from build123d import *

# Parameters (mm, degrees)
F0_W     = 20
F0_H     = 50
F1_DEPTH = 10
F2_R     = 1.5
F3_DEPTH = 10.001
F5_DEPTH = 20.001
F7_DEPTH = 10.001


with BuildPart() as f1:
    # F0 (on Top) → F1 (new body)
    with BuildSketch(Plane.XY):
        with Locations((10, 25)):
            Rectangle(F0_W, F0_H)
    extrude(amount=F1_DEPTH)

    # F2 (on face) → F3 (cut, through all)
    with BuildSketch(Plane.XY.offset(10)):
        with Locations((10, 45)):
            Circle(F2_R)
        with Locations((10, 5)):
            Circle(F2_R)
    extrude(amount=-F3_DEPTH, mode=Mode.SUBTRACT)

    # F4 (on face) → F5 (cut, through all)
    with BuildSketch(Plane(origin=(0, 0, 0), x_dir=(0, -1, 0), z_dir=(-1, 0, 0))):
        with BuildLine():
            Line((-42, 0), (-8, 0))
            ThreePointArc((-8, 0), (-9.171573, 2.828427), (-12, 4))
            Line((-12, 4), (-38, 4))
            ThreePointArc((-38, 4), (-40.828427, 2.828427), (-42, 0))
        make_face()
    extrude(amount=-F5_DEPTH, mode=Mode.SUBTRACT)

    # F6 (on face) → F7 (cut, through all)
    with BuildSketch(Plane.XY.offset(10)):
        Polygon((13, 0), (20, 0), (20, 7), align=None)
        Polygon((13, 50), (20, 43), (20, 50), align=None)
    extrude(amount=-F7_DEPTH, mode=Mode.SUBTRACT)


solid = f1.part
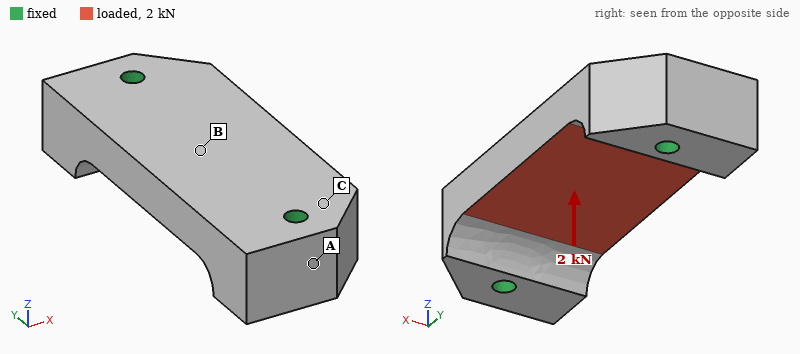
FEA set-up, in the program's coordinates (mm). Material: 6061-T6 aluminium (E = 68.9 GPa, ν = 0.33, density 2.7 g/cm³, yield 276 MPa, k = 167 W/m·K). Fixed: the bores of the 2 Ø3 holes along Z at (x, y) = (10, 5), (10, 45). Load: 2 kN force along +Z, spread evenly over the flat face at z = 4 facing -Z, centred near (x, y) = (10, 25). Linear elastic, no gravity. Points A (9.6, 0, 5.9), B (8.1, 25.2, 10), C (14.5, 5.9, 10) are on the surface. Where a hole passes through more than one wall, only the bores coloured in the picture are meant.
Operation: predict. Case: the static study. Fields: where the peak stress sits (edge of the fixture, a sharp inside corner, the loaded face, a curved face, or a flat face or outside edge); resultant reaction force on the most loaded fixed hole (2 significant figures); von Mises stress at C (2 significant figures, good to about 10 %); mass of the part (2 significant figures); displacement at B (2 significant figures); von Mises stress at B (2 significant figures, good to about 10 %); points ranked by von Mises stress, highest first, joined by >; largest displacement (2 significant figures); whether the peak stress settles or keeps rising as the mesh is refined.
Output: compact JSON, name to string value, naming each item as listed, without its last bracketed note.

{"where the peak stress sits": "edge of the fixture", "resultant reaction force on the most loaded fixed hole": "1.0 kN", "von Mises stress at C": "22 MPa", "mass of the part": "18 g", "displacement at B": "19 µm", "von Mises stress at B": "36 MPa", "points ranked by von Mises stress, highest first, joined by >": "B > C > A", "largest displacement": "22 µm", "whether the peak stress settles or keeps rising as the mesh is refined": "keeps rising"}
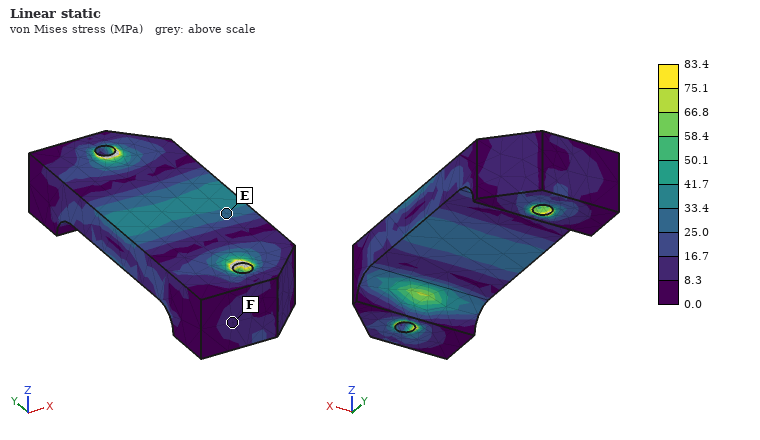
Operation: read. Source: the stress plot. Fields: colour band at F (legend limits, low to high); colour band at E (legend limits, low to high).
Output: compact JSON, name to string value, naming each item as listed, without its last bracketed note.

{"colour band at F": "8.3 to 16.7 MPa", "colour band at E": "25.0 to 33.4 MPa"}
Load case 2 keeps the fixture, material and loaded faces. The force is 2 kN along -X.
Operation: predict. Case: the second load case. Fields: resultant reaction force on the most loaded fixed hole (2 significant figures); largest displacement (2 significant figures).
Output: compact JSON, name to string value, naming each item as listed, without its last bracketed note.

{"resultant reaction force on the most loaded fixed hole": "1.0 kN", "largest displacement": "15 µm"}
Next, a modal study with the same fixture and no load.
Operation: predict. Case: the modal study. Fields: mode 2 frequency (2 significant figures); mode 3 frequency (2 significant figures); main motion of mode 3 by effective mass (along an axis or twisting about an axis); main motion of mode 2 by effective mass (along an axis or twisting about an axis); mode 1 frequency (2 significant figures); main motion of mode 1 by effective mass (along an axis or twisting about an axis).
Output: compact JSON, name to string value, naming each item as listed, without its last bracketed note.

{"mode 2 frequency": "23 kHz", "mode 3 frequency": "25 kHz", "main motion of mode 3 by effective mass": "along X", "main motion of mode 2 by effective mass": "along X", "mode 1 frequency": "19 kHz", "main motion of mode 1 by effective mass": "along Z"}
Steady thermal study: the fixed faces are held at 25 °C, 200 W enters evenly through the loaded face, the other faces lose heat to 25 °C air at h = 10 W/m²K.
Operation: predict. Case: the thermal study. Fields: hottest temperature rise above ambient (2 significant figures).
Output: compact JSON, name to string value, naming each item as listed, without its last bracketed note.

{"hottest temperature rise above ambient": "74 K"}
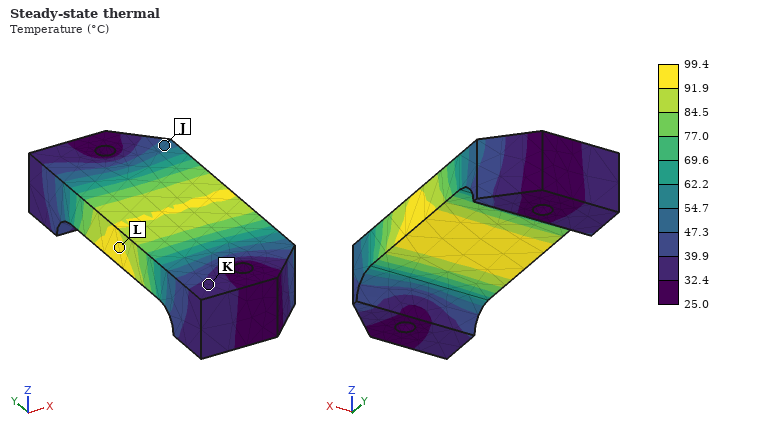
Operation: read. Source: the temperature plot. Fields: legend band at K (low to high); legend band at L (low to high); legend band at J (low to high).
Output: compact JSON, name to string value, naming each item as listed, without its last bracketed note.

{"legend band at K": "32.4 to 39.9 °C", "legend band at L": "91.9 to 99.4 °C", "legend band at J": "47.3 to 54.7 °C"}
